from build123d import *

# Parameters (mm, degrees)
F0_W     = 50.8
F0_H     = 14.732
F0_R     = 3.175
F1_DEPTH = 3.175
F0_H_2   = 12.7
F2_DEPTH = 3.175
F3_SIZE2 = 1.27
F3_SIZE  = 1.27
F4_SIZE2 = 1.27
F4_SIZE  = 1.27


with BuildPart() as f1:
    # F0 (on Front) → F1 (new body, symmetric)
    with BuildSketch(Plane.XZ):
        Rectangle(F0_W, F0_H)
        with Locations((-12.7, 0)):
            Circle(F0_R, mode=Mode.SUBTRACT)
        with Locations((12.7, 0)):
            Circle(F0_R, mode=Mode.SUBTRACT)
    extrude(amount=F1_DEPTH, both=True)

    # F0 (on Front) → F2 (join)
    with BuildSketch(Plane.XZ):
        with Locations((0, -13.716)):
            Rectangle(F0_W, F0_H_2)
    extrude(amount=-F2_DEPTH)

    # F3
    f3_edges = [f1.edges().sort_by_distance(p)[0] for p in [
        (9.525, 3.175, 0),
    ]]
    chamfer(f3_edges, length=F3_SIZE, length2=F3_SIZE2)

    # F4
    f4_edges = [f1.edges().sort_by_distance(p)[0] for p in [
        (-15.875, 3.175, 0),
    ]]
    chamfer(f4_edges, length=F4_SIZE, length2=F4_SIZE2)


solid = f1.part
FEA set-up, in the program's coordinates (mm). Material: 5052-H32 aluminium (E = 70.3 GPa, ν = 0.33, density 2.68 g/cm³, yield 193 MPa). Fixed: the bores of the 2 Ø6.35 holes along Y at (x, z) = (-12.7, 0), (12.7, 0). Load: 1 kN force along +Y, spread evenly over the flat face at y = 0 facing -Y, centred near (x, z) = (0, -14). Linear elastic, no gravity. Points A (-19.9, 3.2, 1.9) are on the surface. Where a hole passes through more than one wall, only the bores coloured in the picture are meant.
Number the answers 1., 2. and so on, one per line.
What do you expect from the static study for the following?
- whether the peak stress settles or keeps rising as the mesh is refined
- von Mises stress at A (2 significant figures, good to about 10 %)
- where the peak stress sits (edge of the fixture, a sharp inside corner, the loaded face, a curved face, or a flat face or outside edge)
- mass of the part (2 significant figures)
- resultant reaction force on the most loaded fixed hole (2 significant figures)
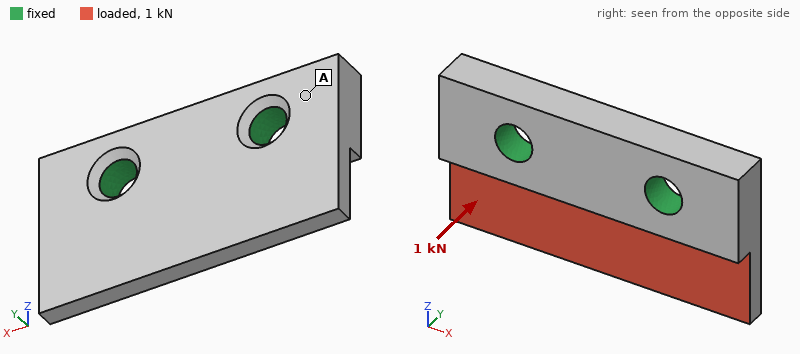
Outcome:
1. keeps rising
2. 13 MPa
3. edge of the fixture
4. 17 g
5. 500 N
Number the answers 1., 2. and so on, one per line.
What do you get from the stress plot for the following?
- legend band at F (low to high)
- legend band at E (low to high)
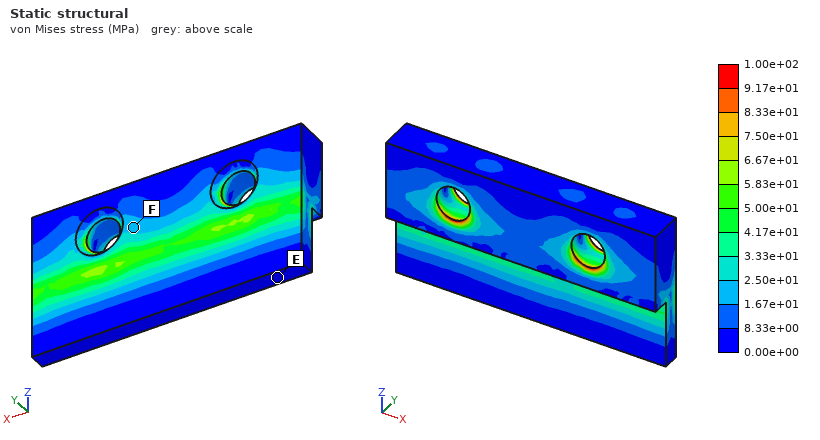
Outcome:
1. 1.67e+01 to 2.50e+01 MPa
2. 0.00e+00 to 8.33e+00 MPa
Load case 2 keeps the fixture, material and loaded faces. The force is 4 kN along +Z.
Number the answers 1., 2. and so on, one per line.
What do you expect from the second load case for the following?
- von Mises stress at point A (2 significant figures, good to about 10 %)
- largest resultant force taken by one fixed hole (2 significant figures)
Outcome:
1. 10 MPa
2. 2.0 kN
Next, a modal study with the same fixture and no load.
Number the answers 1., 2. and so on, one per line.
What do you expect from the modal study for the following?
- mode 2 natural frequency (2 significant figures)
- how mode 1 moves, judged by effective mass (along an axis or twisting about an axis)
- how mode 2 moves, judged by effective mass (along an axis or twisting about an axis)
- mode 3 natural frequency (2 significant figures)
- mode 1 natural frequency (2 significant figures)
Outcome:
1. 13 kHz
2. along Y
3. twisting about Z
4. 17 kHz
5. 11 kHz
